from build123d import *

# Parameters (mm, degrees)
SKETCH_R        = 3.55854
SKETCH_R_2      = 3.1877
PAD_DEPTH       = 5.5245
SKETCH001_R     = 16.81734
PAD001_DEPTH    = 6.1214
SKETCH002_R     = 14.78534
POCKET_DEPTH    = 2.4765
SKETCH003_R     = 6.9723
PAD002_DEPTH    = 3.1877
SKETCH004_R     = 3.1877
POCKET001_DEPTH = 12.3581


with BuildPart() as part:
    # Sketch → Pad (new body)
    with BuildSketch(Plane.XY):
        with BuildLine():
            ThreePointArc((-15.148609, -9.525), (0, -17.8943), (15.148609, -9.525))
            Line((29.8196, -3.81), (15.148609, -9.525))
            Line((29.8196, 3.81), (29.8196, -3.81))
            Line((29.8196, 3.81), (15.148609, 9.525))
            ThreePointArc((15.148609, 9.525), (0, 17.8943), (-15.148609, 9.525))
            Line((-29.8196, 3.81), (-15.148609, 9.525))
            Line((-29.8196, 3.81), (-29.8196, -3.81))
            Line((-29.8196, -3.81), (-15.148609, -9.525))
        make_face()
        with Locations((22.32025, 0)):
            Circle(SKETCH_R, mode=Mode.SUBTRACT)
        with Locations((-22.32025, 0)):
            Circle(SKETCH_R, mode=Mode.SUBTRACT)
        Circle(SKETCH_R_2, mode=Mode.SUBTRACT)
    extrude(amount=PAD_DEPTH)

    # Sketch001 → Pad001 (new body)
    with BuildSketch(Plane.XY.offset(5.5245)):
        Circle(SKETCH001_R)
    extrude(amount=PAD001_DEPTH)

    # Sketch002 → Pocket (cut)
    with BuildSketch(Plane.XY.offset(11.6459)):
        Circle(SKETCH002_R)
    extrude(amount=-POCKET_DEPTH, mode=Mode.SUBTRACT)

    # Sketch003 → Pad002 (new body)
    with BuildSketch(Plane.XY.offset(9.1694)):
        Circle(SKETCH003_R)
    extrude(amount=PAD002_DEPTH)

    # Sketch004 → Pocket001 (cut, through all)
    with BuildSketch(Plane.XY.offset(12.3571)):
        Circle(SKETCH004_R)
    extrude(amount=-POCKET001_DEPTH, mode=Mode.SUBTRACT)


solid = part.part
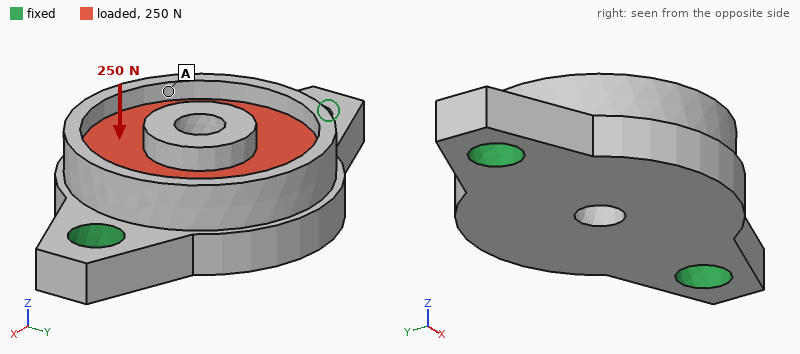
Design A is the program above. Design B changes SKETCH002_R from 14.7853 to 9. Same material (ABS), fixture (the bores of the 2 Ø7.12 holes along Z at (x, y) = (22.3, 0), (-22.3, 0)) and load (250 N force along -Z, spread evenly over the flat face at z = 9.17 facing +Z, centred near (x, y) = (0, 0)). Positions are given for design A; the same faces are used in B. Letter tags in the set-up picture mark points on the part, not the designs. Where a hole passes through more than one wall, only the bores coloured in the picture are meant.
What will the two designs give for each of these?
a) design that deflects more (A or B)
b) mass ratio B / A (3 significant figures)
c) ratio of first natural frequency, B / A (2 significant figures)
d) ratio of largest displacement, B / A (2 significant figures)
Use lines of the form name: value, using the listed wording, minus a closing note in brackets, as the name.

design that deflects more: A
mass ratio B / A: 1.10
ratio of first natural frequency, B / A: 0.95
ratio of largest displacement, B / A: 0.81
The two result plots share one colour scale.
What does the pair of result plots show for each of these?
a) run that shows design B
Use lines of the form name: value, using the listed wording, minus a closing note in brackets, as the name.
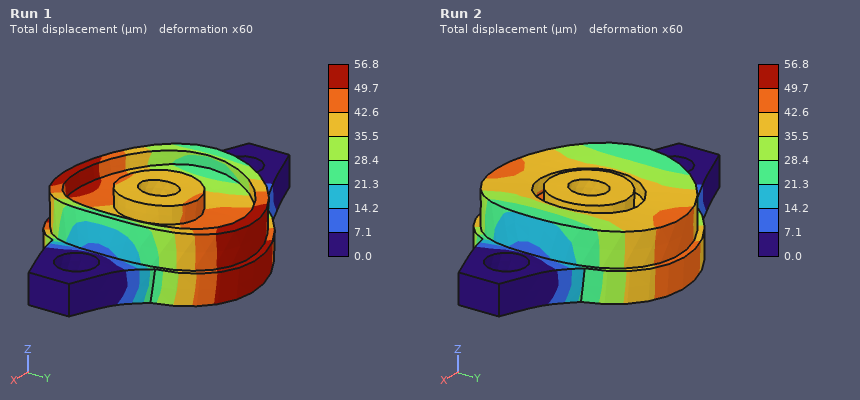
run that shows design B: Run 2
